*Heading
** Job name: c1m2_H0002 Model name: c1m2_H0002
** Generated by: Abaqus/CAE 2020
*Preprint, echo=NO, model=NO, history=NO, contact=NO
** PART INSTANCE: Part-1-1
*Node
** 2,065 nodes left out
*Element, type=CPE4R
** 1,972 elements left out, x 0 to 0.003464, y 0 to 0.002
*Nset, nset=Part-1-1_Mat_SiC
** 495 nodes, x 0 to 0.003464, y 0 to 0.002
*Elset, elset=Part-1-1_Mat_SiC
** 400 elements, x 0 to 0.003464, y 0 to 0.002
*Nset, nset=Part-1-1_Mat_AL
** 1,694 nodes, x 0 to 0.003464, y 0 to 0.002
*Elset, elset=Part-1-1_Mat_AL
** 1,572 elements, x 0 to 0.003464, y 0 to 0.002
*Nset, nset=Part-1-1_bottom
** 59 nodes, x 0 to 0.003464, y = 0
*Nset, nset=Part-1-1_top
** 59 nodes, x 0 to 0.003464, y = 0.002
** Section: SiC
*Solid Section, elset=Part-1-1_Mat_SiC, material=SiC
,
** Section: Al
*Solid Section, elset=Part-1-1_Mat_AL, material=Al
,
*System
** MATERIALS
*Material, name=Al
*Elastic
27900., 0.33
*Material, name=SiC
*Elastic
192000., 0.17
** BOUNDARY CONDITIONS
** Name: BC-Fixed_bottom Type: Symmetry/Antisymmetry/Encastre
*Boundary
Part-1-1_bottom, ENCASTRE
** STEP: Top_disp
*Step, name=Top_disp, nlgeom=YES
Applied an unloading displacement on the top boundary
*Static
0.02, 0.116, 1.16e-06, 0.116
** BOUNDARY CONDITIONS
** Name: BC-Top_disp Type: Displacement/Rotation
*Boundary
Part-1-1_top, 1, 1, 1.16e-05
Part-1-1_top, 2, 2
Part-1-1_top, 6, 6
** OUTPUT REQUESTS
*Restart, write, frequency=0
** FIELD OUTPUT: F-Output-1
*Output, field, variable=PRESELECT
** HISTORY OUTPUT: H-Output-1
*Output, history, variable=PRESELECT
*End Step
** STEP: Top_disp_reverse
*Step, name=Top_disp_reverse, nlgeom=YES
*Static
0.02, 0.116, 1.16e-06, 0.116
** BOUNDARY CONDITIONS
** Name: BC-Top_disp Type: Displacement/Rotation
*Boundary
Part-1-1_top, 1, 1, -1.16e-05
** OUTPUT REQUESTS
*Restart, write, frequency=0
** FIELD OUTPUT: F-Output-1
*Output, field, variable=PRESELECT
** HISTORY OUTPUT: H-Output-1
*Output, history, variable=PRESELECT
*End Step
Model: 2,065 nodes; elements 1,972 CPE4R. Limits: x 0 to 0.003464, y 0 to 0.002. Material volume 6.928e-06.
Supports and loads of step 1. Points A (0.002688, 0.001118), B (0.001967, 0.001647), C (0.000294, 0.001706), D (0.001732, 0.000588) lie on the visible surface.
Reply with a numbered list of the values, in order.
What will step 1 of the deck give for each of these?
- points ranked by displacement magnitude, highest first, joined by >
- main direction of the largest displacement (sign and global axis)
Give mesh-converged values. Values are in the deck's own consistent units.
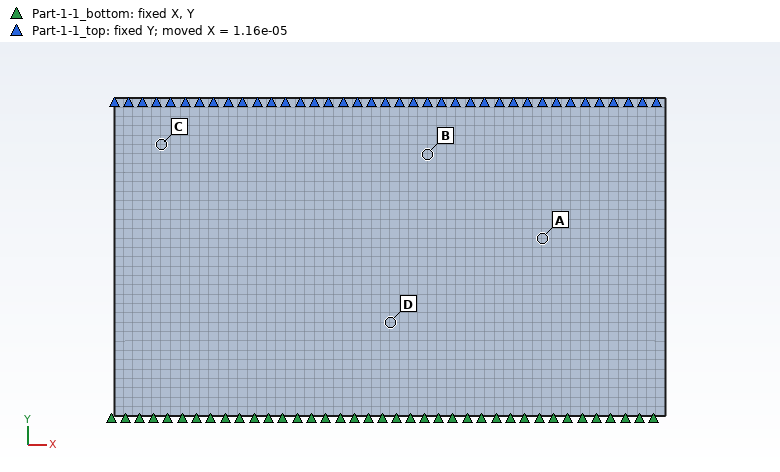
1. C > B > A > D
2. +X
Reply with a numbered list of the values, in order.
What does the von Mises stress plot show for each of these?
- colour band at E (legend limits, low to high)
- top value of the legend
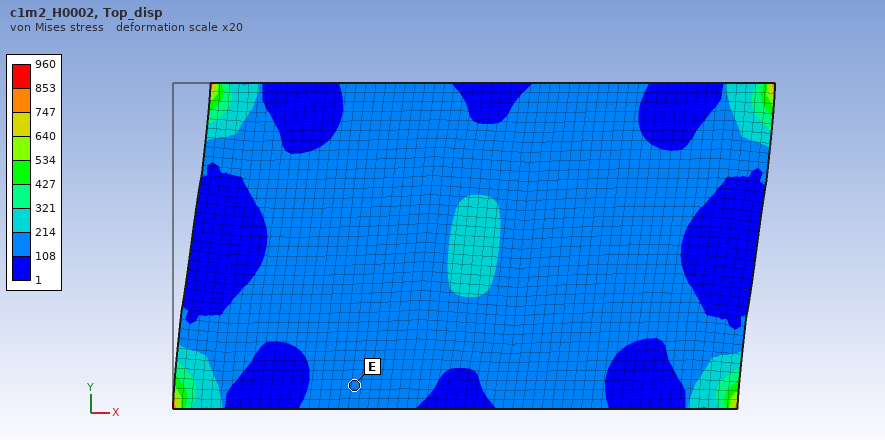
1. 108 to 214
2. 960
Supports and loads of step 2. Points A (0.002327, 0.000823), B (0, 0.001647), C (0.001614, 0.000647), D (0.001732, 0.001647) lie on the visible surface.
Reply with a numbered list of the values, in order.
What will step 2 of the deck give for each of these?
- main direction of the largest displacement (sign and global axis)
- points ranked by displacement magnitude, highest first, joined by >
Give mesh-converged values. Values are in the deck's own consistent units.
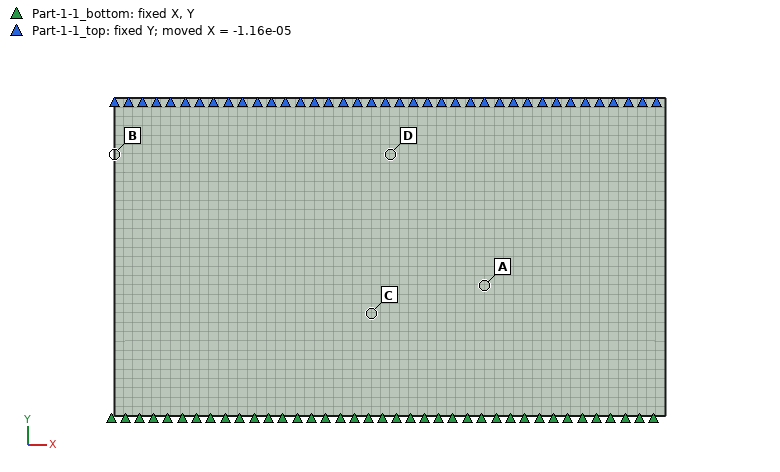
1. -X
2. B > D > A > C
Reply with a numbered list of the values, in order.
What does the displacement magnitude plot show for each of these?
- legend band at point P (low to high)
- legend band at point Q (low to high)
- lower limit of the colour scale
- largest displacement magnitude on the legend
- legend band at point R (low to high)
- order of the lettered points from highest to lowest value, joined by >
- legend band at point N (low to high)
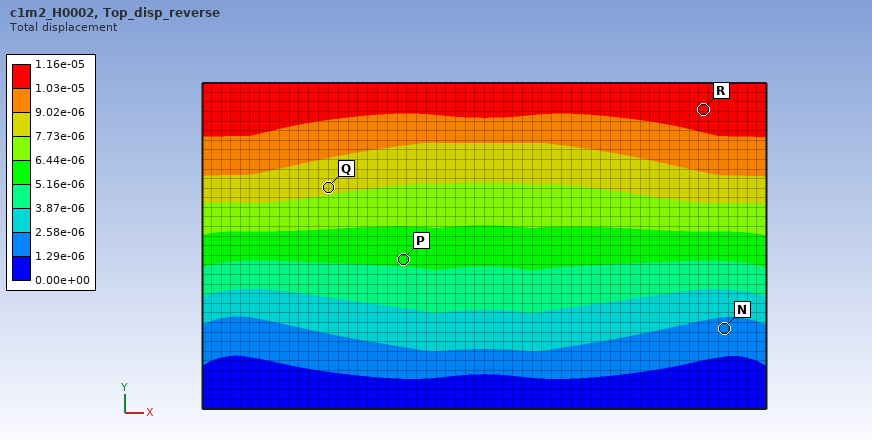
1. 5.16e-06 to 6.44e-06
2. 7.73e-06 to 9.02e-06
3. 0.00e+00
4. 1.16e-05
5. 1.03e-05 to 1.16e-05
6. R > Q > P > N
7. 1.29e-06 to 2.58e-06
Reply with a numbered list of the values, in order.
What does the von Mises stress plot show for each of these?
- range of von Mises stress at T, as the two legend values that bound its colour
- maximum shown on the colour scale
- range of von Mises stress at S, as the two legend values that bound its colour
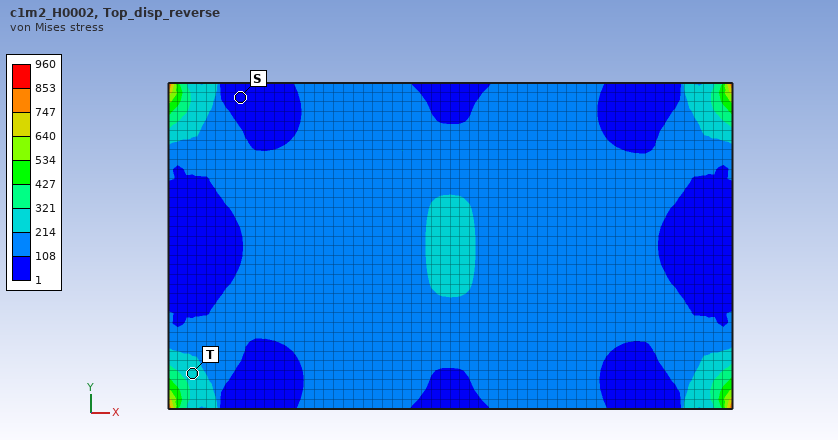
1. 214 to 321
2. 960
3. 1 to 108
